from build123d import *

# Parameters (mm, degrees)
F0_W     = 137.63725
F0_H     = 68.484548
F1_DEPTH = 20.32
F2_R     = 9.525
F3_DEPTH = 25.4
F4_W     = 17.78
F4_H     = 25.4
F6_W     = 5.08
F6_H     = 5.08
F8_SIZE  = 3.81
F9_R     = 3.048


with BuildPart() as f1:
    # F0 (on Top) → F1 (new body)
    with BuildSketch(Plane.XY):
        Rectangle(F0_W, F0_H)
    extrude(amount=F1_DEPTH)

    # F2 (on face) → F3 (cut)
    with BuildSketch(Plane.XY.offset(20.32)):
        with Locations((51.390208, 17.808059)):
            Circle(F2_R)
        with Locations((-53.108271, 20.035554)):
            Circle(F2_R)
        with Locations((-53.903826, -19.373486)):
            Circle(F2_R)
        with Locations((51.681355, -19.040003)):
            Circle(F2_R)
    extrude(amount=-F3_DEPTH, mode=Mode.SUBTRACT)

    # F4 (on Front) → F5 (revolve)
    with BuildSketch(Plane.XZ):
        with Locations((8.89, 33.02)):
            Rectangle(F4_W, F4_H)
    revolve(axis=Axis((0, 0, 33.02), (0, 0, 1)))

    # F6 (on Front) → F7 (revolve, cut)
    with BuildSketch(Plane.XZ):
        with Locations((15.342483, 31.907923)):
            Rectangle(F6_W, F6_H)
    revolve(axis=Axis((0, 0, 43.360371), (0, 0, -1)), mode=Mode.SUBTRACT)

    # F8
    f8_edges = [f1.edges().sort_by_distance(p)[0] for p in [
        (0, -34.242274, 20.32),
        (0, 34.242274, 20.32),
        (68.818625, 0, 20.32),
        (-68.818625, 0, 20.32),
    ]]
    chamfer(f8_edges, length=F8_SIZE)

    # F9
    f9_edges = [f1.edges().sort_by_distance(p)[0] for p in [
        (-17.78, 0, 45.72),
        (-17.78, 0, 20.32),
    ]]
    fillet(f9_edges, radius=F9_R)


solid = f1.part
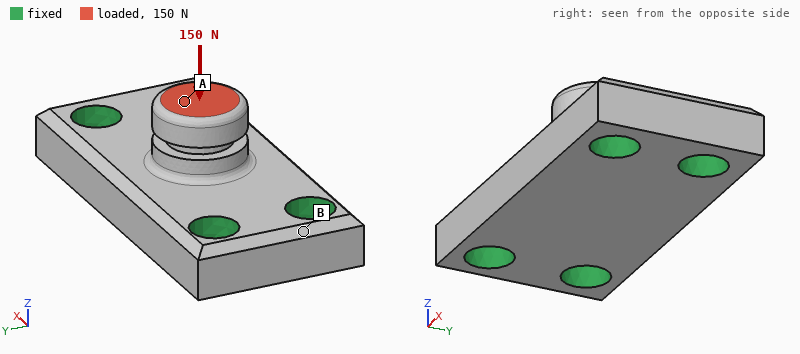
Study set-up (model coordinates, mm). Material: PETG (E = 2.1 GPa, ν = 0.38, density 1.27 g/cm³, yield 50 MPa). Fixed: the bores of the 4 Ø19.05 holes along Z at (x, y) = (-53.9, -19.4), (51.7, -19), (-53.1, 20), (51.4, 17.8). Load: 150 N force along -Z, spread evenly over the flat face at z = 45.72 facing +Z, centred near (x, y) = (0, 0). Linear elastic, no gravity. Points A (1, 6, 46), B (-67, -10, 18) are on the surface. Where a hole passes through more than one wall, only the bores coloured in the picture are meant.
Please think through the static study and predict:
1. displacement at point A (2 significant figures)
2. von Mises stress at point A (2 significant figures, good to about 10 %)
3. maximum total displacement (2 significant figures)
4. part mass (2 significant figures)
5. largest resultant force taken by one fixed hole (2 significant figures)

9.3 µm
0.24 MPa
9.6 µm
240 g
41 N
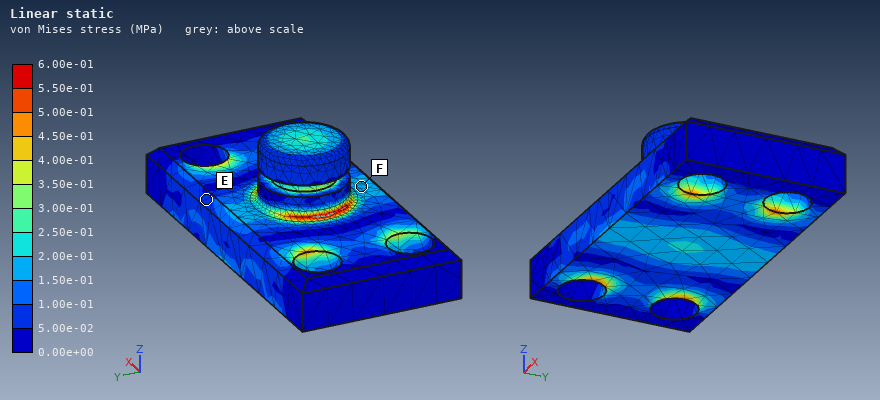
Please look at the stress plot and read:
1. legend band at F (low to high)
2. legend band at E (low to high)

1.50e-01 to 2.00e-01 MPa
5.00e-02 to 1.00e-01 MPa
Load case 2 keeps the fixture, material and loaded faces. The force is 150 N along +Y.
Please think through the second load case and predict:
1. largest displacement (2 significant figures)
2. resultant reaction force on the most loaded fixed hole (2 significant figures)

44 µm
77 N
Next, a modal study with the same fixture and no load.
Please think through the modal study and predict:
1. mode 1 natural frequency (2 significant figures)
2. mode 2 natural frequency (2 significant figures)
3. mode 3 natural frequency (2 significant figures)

2200 Hz
2300 Hz
3300 Hz
